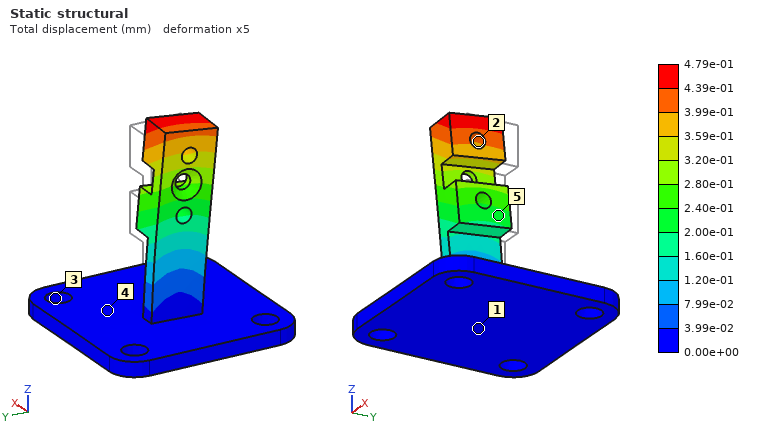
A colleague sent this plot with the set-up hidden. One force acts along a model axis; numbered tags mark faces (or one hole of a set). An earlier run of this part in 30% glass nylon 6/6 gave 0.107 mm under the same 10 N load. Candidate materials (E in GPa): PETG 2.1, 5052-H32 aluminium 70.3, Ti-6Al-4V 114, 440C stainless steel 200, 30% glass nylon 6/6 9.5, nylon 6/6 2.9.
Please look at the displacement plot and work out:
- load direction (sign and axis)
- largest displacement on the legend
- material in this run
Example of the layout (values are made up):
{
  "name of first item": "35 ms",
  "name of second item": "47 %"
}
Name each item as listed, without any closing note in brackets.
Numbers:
{
  "load direction": "-Y",
  "largest displacement on the legend": "4.79e-01 mm",
  "material in this run": "PETG"
}
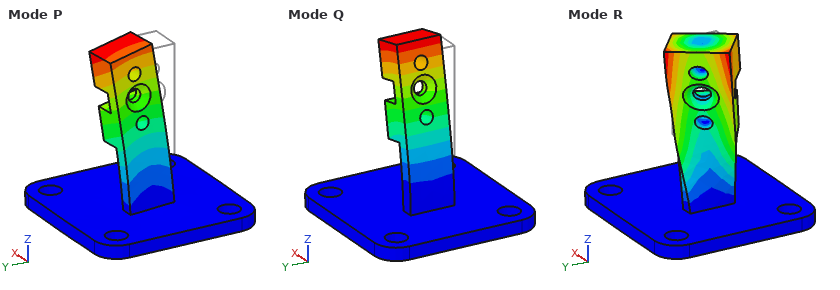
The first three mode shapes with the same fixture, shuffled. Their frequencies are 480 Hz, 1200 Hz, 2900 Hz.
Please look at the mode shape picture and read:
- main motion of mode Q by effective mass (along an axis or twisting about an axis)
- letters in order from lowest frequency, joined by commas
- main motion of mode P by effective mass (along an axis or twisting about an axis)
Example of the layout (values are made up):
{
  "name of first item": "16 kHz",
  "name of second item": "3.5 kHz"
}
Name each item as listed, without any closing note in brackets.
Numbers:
{
  "main motion of mode Q by effective mass": "along X",
  "letters in order from lowest frequency, joined by commas": "Q, P, R",
  "main motion of mode P by effective mass": "along Y"
}
